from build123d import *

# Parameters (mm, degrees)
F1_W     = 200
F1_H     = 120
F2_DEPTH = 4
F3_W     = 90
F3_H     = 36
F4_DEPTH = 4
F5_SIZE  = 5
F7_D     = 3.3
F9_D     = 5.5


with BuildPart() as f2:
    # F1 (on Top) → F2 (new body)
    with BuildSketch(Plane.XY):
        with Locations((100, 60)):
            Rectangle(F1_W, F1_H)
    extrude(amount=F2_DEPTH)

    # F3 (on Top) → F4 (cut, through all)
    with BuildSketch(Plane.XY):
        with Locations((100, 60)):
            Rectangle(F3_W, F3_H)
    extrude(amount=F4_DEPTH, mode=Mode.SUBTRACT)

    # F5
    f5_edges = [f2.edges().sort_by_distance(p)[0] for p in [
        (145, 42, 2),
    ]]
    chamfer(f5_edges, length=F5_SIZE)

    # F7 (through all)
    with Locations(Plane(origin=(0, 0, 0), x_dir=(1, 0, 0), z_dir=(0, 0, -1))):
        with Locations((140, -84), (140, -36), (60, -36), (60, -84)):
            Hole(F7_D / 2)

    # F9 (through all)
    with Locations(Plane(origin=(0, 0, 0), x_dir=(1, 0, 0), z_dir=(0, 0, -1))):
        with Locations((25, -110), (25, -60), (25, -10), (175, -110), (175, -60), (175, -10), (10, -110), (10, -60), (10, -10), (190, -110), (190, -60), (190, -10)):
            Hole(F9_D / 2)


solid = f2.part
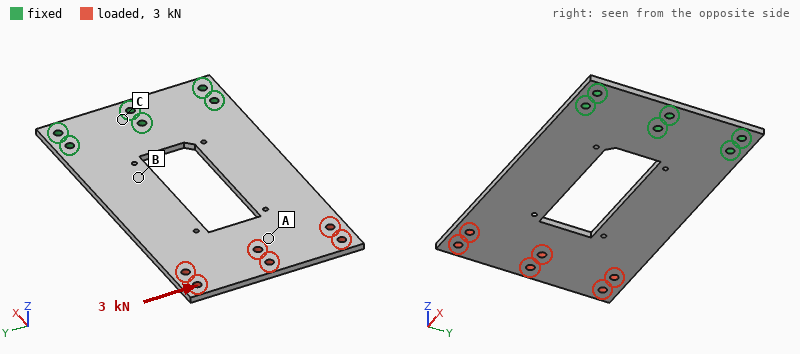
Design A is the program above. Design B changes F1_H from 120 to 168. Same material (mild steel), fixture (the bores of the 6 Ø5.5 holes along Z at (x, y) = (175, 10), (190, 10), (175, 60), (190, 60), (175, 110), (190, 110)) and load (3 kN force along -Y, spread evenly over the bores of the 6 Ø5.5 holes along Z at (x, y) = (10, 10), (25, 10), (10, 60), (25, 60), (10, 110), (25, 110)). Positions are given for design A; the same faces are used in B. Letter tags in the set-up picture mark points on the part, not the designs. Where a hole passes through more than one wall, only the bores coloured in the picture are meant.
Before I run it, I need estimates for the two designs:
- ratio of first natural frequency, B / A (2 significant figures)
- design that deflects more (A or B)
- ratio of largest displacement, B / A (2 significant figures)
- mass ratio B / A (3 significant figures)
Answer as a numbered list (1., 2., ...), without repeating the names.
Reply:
1. 1.0
2. A
3. 0.58
4. 1.47
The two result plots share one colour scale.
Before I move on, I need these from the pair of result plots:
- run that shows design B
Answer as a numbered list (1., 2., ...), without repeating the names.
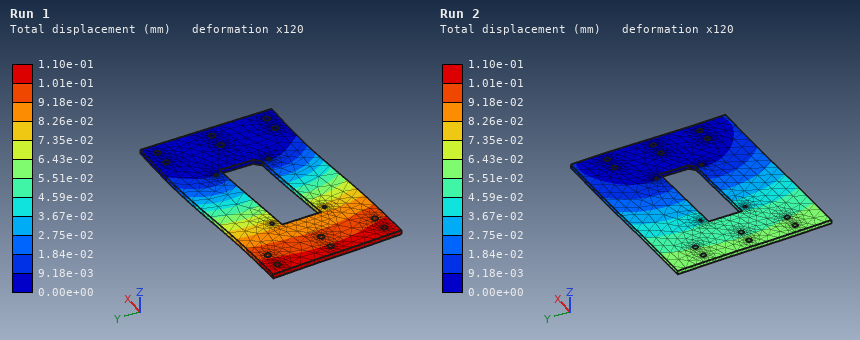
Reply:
1. Run 2
